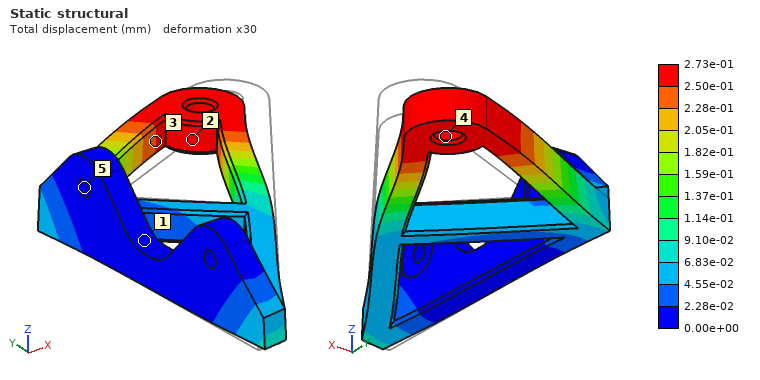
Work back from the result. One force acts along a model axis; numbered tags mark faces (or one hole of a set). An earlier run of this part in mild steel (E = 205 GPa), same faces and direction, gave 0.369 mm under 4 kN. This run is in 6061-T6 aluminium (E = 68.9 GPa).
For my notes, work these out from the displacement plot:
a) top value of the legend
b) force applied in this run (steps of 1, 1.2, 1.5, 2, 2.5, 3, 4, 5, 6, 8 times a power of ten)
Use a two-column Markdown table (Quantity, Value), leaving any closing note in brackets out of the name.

| Quantity | Value |
|---|---|
| top value of the legend | 2.73e-01 mm |
| force applied in this run | 1 kN |
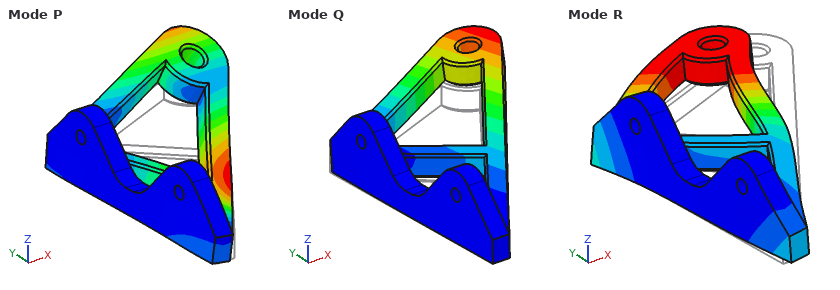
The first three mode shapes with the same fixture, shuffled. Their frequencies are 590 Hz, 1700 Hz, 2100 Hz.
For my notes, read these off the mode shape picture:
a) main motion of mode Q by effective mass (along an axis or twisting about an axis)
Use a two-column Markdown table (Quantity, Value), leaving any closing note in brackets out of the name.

| Quantity | Value |
|---|---|
| main motion of mode Q by effective mass | along Z |
